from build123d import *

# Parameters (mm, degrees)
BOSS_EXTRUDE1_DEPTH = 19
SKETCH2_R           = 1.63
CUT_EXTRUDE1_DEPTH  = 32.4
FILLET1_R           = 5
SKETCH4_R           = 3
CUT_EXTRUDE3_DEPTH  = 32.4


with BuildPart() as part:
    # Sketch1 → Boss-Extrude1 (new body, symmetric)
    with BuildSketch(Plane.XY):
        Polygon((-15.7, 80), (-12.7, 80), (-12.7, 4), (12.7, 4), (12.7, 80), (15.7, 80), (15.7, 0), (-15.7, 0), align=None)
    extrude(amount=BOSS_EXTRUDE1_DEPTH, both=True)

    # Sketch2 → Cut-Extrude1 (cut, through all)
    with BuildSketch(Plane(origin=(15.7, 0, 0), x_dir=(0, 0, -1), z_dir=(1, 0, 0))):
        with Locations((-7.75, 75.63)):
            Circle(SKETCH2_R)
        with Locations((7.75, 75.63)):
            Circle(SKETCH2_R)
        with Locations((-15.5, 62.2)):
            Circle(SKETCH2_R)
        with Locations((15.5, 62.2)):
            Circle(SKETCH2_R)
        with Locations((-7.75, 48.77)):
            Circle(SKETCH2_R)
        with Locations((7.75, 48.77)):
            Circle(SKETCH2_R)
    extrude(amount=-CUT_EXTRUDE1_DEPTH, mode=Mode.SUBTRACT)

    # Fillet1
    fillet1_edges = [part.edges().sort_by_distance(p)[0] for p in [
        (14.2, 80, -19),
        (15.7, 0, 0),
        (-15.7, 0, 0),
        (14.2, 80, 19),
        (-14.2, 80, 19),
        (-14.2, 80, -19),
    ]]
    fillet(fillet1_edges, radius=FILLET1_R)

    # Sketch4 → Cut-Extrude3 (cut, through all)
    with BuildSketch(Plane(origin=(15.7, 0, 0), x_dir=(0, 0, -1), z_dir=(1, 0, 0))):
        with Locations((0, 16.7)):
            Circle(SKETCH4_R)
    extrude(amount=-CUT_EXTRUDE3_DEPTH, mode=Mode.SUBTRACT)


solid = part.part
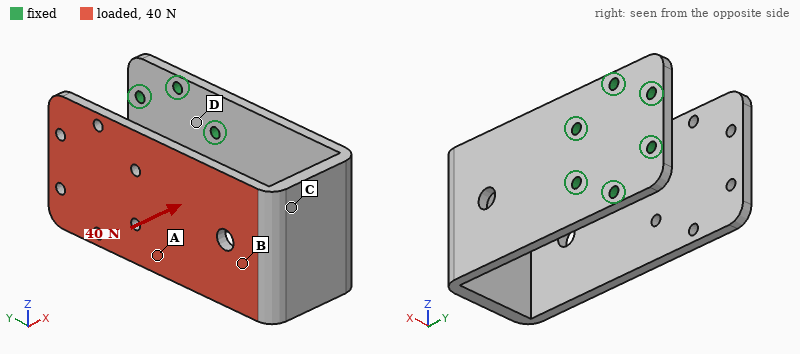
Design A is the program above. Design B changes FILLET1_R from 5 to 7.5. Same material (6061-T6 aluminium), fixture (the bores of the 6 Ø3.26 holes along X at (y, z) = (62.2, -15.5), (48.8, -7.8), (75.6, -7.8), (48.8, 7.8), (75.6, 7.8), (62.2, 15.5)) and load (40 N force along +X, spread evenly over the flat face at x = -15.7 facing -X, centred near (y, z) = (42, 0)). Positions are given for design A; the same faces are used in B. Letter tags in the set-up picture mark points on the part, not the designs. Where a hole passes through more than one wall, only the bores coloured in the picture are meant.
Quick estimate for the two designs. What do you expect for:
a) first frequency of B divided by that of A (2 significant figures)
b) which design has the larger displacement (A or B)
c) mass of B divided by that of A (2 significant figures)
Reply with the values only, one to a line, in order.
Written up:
0.94
B
0.97
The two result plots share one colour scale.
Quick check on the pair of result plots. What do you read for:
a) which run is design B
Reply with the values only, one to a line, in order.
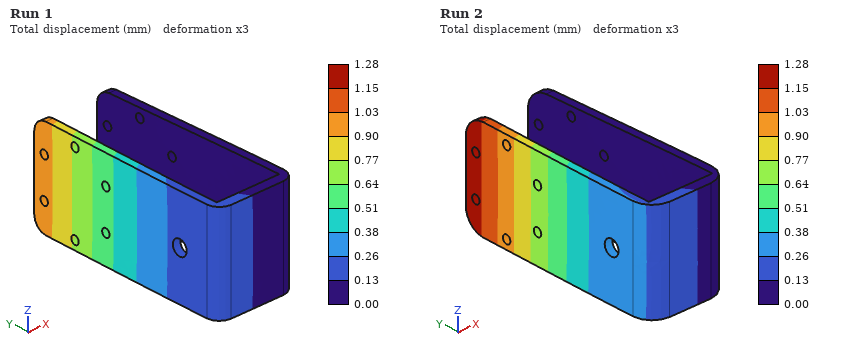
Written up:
Run 2
